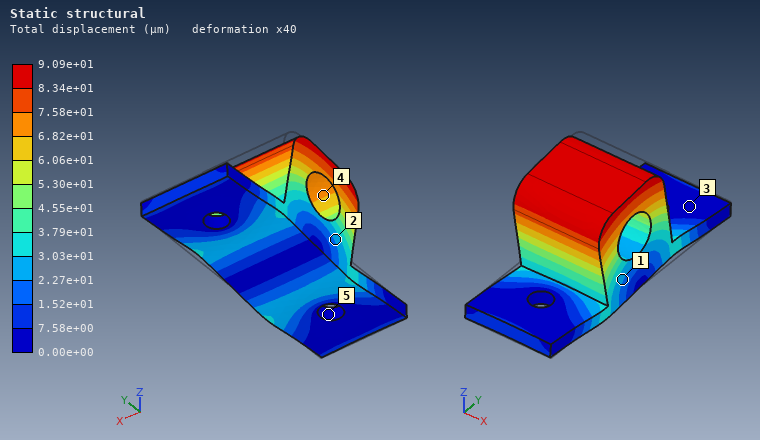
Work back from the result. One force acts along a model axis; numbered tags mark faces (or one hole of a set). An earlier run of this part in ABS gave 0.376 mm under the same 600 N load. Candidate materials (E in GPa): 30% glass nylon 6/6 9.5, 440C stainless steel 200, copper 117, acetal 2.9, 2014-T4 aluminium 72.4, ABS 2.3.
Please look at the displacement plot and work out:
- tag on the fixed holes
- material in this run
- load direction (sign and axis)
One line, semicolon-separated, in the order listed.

5; 30% glass nylon 6/6; -Y
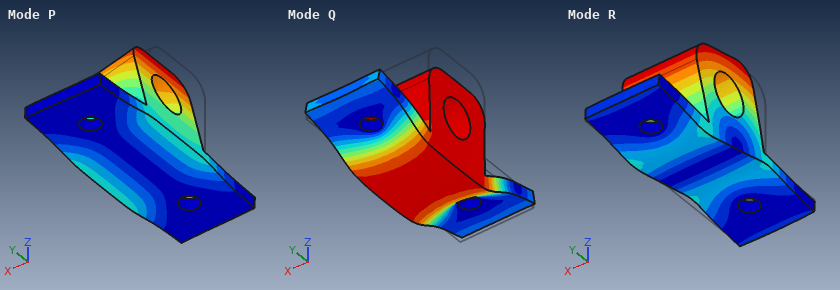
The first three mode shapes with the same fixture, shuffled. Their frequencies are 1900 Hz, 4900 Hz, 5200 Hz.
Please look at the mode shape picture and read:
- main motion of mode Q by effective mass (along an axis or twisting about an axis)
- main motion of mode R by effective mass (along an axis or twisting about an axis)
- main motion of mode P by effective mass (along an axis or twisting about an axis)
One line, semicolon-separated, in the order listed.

along Z; along Y; along X
